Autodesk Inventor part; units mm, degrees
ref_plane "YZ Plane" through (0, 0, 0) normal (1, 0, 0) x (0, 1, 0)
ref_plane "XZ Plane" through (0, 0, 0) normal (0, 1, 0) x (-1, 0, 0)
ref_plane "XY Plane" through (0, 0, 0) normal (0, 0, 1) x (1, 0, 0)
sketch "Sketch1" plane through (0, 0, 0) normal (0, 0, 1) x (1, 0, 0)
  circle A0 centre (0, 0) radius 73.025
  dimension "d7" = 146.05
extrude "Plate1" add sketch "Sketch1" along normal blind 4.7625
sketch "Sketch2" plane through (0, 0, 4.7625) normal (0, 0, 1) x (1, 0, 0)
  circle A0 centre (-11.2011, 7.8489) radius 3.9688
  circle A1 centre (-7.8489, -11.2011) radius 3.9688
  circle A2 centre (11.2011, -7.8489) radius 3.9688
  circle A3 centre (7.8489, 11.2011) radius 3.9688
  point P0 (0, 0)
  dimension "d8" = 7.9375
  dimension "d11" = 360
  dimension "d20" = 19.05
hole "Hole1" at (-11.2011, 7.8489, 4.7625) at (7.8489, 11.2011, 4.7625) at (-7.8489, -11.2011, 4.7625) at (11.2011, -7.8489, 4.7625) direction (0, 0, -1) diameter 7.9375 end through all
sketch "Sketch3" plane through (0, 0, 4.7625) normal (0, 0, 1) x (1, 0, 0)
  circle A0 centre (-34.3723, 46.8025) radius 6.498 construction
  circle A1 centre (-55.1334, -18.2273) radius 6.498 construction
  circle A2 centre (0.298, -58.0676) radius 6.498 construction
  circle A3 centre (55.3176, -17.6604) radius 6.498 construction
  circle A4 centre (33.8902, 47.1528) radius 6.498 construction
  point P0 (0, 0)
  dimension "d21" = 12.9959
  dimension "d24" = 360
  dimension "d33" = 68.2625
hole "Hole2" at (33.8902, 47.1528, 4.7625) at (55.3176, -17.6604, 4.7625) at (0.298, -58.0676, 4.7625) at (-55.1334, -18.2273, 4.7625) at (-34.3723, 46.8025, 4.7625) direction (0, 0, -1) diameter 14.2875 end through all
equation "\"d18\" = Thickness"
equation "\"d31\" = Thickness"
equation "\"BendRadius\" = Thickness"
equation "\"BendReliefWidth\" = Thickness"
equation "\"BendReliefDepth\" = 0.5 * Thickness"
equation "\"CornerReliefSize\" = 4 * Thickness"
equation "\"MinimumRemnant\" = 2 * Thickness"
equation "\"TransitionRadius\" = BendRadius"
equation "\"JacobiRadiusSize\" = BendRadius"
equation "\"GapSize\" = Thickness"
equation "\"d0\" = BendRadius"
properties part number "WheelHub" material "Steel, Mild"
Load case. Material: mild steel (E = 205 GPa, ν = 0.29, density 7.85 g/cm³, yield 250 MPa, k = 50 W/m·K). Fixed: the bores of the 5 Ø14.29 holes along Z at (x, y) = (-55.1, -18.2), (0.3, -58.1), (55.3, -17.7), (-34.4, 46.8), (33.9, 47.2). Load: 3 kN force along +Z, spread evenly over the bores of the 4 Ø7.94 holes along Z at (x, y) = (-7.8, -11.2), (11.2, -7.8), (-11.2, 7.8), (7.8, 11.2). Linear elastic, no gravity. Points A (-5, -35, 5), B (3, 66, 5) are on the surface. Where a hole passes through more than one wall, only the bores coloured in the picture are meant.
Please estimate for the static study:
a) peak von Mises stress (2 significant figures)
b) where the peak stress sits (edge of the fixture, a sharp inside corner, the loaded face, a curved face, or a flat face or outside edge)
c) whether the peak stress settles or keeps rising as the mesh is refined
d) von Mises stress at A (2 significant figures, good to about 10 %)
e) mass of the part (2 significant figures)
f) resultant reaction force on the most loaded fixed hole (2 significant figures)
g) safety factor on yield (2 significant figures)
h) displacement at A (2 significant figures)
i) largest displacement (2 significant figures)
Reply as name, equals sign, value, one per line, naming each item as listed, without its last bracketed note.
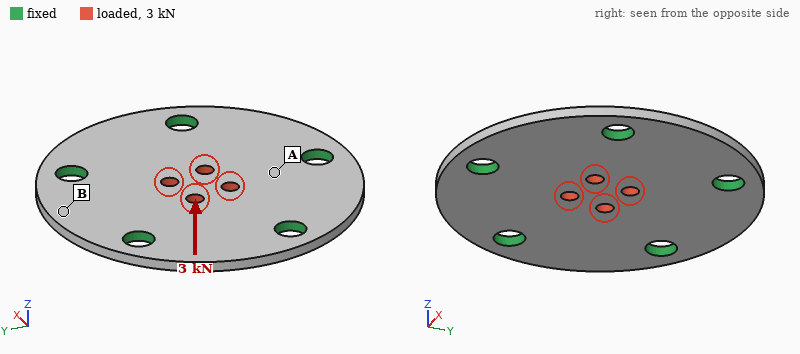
peak von Mises stress = 180 MPa
where the peak stress sits = the loaded face
whether the peak stress settles or keeps rising as the mesh is refined = settles
von Mises stress at A = 33 MPa
mass of the part = 590 g
resultant reaction force on the most loaded fixed hole = 600 N
safety factor on yield = 1.4
displacement at A = 25 µm
largest displacement = 89 µm
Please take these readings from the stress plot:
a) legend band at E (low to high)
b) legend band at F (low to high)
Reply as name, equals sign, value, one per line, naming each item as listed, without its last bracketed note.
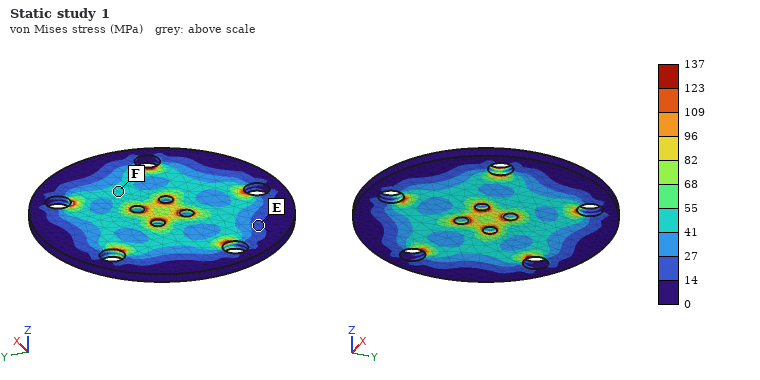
legend band at E = 14 to 27 MPa
legend band at F = 41 to 55 MPa
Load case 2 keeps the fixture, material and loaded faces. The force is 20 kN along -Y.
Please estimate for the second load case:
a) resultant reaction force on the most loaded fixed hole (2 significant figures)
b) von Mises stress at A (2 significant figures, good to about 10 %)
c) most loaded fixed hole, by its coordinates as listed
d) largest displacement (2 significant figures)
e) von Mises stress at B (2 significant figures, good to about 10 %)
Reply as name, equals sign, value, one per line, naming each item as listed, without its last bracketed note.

resultant reaction force on the most loaded fixed hole = 5.9 kN
von Mises stress at A = 43 MPa
most loaded fixed hole, by its coordinates as listed = (0.3, -58.1)
largest displacement = 11 µm
von Mises stress at B = 12 MPa
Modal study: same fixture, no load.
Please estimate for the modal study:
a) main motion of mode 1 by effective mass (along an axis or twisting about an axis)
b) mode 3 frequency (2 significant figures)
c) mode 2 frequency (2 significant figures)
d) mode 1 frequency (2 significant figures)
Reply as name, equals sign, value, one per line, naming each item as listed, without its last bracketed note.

main motion of mode 1 by effective mass = along Z
mode 3 frequency = 5400 Hz
mode 2 frequency = 5400 Hz
mode 1 frequency = 3500 Hz
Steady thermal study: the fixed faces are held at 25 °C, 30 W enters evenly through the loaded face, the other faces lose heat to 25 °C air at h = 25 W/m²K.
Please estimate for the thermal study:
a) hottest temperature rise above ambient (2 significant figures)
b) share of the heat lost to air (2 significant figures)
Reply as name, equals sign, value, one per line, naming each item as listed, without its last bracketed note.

hottest temperature rise above ambient = 33 K
share of the heat lost to air = 19 %
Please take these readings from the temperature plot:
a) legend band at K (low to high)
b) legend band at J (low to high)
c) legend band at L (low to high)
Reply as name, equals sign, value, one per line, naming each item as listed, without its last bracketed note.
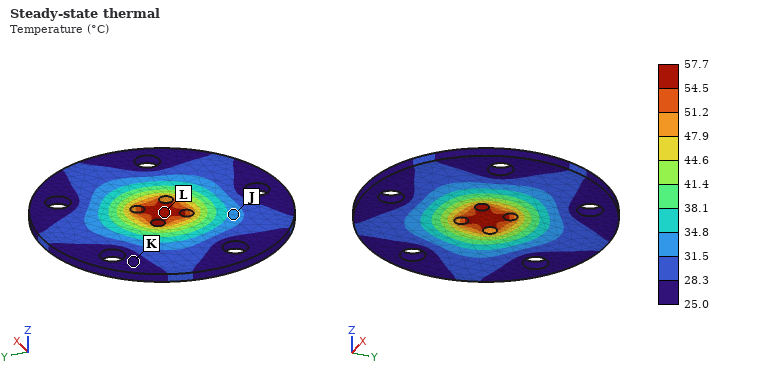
legend band at K = 25.0 to 28.3 °C
legend band at J = 31.5 to 34.8 °C
legend band at L = 54.5 to 57.7 °C
